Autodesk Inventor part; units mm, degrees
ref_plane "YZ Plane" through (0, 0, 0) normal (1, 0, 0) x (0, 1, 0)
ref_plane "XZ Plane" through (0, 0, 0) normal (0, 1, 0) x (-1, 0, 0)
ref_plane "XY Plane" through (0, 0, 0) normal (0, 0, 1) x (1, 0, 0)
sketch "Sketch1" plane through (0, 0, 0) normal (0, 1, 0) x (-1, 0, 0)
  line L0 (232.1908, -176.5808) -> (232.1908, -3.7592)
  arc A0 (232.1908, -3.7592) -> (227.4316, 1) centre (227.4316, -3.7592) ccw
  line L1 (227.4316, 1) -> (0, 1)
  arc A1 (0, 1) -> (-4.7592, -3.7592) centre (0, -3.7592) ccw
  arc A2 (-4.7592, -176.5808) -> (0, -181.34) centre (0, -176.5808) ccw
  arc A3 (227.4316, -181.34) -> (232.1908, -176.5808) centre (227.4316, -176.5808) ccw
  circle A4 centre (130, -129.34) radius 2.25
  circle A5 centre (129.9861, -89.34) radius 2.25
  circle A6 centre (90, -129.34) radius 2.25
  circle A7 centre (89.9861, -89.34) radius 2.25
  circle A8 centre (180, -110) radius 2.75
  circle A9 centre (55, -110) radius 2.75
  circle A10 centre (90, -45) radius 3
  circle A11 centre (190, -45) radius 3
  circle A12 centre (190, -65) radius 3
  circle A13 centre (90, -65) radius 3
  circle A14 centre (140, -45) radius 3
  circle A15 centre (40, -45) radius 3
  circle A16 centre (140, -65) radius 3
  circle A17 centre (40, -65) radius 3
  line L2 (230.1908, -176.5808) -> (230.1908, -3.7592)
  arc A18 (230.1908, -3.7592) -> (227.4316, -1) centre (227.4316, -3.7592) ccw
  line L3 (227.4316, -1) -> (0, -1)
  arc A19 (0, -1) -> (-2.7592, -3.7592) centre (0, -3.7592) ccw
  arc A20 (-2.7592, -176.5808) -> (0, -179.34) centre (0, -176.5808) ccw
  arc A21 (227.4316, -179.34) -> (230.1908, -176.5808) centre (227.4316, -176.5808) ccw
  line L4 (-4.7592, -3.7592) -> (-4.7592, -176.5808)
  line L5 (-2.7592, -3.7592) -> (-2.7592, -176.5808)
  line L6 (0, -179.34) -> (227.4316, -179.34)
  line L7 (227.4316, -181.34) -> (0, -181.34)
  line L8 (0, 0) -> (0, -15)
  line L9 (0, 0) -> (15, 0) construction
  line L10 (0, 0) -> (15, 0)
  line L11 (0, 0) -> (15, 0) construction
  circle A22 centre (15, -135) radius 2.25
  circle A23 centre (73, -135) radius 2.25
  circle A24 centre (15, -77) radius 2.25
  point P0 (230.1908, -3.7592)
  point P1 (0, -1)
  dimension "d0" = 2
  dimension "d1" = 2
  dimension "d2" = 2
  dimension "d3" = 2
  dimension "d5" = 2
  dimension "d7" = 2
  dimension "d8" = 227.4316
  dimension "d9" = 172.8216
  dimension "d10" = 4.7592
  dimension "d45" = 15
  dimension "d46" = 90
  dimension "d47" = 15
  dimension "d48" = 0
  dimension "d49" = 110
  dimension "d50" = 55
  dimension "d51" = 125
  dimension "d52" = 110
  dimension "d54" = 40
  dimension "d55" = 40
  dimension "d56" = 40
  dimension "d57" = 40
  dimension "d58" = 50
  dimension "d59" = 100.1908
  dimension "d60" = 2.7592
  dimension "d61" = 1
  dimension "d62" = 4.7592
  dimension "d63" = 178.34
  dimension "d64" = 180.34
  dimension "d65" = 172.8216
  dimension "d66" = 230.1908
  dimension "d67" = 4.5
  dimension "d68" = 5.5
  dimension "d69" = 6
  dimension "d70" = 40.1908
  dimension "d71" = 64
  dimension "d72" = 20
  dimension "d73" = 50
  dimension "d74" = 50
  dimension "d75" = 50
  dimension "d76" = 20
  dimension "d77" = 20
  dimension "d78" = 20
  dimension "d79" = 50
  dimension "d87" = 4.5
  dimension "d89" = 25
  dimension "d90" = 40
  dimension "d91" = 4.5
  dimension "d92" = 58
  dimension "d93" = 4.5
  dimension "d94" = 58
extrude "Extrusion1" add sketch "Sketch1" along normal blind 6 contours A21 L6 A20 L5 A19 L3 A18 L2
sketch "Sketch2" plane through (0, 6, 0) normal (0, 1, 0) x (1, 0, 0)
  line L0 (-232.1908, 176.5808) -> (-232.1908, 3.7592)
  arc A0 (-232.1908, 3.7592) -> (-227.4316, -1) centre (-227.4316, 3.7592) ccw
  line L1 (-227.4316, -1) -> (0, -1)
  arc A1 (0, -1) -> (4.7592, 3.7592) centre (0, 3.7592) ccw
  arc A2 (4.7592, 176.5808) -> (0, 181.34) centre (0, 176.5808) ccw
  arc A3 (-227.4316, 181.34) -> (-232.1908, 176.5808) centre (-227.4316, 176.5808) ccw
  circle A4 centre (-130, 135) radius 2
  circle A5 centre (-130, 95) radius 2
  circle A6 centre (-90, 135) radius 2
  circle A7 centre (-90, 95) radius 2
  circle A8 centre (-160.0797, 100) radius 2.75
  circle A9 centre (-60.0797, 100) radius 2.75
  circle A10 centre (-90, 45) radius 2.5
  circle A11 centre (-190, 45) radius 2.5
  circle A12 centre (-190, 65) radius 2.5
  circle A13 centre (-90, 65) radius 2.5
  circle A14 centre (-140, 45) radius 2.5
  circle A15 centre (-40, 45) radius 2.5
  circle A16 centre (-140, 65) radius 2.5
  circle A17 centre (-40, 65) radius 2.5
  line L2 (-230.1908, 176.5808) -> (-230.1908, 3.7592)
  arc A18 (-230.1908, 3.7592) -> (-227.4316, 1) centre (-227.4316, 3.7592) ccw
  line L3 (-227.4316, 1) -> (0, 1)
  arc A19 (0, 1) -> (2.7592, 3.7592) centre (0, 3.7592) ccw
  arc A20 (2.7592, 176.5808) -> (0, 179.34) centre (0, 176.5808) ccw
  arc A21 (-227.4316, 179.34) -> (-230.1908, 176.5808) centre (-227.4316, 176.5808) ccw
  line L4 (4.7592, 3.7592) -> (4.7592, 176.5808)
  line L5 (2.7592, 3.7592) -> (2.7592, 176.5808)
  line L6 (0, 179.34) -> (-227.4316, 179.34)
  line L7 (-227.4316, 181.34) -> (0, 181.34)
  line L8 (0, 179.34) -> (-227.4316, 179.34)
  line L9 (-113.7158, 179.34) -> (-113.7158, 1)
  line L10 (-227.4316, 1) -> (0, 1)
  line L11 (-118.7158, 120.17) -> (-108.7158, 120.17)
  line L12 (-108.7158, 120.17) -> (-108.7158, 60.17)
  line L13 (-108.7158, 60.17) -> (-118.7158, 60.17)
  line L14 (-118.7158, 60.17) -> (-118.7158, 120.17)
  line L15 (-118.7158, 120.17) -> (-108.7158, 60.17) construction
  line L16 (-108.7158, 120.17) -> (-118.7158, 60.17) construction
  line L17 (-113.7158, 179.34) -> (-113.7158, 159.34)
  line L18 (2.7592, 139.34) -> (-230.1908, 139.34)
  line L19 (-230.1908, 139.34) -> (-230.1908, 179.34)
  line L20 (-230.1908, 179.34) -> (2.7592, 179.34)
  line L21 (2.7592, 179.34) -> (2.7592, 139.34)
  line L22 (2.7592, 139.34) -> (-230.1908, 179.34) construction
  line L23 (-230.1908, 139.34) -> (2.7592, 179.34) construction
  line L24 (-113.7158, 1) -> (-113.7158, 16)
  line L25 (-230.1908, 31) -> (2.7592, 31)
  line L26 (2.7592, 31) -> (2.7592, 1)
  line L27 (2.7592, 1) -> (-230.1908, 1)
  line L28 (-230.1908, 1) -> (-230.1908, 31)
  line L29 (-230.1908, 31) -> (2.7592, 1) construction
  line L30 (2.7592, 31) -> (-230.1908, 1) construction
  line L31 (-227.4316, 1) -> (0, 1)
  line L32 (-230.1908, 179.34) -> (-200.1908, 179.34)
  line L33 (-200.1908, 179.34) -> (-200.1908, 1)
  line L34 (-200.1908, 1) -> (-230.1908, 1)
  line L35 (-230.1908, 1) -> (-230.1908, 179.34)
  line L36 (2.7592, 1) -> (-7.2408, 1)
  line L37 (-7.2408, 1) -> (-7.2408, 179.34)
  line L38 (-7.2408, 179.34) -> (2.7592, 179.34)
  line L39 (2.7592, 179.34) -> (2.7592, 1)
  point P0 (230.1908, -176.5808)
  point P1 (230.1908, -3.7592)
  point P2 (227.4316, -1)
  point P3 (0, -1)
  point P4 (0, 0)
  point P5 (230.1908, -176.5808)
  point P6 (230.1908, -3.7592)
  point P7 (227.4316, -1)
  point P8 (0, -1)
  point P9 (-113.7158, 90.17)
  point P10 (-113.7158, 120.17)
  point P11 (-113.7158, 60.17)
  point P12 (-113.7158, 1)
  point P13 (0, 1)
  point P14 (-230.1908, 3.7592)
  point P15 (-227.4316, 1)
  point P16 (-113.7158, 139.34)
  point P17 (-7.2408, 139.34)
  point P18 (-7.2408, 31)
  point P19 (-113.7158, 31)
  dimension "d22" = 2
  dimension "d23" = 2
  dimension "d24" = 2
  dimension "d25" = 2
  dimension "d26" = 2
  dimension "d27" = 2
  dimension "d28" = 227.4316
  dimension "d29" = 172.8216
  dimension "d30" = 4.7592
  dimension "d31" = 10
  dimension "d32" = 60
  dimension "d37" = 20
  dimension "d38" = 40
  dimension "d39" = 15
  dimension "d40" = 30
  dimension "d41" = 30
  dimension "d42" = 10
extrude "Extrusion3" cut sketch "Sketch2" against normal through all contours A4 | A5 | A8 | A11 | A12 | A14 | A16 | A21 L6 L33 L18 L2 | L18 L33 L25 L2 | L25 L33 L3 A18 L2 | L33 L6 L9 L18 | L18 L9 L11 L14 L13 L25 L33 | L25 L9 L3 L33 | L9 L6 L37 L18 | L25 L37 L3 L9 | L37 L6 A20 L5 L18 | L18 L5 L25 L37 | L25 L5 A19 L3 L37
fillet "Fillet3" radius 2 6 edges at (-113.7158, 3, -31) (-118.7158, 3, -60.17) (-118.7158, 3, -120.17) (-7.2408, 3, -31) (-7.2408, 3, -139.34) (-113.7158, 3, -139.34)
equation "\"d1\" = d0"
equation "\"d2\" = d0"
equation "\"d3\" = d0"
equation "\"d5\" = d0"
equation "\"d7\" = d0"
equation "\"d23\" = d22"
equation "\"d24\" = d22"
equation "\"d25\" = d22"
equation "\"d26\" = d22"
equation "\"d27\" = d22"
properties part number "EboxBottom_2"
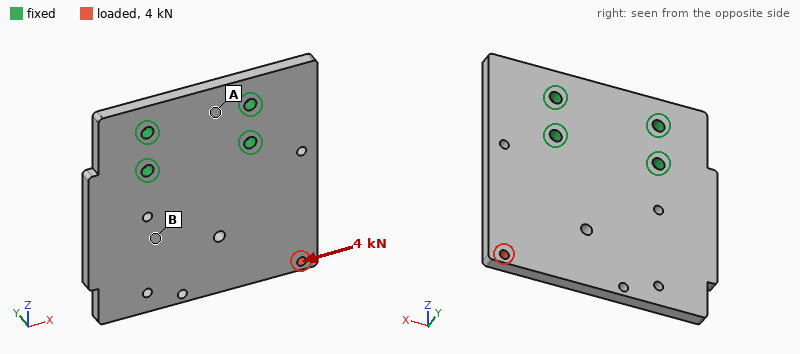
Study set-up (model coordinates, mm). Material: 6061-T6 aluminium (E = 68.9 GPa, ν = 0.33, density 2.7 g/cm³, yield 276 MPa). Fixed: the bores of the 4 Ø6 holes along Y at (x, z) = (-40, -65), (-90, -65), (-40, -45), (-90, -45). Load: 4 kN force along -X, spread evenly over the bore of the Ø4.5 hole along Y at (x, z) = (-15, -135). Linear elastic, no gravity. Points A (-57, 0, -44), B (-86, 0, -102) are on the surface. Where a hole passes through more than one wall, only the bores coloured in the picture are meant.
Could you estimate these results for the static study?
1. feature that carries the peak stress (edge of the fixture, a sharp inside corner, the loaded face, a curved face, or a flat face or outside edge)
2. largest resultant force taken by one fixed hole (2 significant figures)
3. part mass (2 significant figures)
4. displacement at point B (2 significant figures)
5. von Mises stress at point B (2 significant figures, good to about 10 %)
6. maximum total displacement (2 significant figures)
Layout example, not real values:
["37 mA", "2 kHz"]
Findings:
["the loaded face", "4.2 kN", "190 g", "24 µm", "15 MPa", "86 µm"]
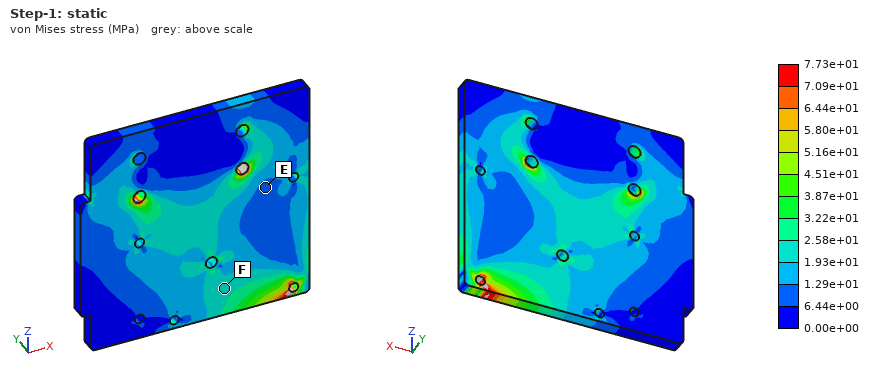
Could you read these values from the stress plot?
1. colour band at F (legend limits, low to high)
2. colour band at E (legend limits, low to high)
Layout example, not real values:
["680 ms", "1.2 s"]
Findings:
["1.93e+01 to 2.58e+01 MPa", "6.44e+00 to 1.29e+01 MPa"]
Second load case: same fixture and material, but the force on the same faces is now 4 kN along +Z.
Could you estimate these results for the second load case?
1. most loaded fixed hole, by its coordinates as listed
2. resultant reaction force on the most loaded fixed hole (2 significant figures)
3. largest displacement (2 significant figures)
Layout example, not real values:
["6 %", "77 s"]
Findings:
["(-40, -65)", "3.7 kN", "56 µm"]
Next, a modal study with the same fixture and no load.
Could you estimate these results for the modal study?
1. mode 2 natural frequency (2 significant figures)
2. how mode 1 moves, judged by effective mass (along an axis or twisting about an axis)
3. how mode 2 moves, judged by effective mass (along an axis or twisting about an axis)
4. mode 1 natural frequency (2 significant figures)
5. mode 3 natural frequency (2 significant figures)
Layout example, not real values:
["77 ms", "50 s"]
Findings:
["1500 Hz", "along Y", "twisting about Z", "870 Hz", "3200 Hz"]
